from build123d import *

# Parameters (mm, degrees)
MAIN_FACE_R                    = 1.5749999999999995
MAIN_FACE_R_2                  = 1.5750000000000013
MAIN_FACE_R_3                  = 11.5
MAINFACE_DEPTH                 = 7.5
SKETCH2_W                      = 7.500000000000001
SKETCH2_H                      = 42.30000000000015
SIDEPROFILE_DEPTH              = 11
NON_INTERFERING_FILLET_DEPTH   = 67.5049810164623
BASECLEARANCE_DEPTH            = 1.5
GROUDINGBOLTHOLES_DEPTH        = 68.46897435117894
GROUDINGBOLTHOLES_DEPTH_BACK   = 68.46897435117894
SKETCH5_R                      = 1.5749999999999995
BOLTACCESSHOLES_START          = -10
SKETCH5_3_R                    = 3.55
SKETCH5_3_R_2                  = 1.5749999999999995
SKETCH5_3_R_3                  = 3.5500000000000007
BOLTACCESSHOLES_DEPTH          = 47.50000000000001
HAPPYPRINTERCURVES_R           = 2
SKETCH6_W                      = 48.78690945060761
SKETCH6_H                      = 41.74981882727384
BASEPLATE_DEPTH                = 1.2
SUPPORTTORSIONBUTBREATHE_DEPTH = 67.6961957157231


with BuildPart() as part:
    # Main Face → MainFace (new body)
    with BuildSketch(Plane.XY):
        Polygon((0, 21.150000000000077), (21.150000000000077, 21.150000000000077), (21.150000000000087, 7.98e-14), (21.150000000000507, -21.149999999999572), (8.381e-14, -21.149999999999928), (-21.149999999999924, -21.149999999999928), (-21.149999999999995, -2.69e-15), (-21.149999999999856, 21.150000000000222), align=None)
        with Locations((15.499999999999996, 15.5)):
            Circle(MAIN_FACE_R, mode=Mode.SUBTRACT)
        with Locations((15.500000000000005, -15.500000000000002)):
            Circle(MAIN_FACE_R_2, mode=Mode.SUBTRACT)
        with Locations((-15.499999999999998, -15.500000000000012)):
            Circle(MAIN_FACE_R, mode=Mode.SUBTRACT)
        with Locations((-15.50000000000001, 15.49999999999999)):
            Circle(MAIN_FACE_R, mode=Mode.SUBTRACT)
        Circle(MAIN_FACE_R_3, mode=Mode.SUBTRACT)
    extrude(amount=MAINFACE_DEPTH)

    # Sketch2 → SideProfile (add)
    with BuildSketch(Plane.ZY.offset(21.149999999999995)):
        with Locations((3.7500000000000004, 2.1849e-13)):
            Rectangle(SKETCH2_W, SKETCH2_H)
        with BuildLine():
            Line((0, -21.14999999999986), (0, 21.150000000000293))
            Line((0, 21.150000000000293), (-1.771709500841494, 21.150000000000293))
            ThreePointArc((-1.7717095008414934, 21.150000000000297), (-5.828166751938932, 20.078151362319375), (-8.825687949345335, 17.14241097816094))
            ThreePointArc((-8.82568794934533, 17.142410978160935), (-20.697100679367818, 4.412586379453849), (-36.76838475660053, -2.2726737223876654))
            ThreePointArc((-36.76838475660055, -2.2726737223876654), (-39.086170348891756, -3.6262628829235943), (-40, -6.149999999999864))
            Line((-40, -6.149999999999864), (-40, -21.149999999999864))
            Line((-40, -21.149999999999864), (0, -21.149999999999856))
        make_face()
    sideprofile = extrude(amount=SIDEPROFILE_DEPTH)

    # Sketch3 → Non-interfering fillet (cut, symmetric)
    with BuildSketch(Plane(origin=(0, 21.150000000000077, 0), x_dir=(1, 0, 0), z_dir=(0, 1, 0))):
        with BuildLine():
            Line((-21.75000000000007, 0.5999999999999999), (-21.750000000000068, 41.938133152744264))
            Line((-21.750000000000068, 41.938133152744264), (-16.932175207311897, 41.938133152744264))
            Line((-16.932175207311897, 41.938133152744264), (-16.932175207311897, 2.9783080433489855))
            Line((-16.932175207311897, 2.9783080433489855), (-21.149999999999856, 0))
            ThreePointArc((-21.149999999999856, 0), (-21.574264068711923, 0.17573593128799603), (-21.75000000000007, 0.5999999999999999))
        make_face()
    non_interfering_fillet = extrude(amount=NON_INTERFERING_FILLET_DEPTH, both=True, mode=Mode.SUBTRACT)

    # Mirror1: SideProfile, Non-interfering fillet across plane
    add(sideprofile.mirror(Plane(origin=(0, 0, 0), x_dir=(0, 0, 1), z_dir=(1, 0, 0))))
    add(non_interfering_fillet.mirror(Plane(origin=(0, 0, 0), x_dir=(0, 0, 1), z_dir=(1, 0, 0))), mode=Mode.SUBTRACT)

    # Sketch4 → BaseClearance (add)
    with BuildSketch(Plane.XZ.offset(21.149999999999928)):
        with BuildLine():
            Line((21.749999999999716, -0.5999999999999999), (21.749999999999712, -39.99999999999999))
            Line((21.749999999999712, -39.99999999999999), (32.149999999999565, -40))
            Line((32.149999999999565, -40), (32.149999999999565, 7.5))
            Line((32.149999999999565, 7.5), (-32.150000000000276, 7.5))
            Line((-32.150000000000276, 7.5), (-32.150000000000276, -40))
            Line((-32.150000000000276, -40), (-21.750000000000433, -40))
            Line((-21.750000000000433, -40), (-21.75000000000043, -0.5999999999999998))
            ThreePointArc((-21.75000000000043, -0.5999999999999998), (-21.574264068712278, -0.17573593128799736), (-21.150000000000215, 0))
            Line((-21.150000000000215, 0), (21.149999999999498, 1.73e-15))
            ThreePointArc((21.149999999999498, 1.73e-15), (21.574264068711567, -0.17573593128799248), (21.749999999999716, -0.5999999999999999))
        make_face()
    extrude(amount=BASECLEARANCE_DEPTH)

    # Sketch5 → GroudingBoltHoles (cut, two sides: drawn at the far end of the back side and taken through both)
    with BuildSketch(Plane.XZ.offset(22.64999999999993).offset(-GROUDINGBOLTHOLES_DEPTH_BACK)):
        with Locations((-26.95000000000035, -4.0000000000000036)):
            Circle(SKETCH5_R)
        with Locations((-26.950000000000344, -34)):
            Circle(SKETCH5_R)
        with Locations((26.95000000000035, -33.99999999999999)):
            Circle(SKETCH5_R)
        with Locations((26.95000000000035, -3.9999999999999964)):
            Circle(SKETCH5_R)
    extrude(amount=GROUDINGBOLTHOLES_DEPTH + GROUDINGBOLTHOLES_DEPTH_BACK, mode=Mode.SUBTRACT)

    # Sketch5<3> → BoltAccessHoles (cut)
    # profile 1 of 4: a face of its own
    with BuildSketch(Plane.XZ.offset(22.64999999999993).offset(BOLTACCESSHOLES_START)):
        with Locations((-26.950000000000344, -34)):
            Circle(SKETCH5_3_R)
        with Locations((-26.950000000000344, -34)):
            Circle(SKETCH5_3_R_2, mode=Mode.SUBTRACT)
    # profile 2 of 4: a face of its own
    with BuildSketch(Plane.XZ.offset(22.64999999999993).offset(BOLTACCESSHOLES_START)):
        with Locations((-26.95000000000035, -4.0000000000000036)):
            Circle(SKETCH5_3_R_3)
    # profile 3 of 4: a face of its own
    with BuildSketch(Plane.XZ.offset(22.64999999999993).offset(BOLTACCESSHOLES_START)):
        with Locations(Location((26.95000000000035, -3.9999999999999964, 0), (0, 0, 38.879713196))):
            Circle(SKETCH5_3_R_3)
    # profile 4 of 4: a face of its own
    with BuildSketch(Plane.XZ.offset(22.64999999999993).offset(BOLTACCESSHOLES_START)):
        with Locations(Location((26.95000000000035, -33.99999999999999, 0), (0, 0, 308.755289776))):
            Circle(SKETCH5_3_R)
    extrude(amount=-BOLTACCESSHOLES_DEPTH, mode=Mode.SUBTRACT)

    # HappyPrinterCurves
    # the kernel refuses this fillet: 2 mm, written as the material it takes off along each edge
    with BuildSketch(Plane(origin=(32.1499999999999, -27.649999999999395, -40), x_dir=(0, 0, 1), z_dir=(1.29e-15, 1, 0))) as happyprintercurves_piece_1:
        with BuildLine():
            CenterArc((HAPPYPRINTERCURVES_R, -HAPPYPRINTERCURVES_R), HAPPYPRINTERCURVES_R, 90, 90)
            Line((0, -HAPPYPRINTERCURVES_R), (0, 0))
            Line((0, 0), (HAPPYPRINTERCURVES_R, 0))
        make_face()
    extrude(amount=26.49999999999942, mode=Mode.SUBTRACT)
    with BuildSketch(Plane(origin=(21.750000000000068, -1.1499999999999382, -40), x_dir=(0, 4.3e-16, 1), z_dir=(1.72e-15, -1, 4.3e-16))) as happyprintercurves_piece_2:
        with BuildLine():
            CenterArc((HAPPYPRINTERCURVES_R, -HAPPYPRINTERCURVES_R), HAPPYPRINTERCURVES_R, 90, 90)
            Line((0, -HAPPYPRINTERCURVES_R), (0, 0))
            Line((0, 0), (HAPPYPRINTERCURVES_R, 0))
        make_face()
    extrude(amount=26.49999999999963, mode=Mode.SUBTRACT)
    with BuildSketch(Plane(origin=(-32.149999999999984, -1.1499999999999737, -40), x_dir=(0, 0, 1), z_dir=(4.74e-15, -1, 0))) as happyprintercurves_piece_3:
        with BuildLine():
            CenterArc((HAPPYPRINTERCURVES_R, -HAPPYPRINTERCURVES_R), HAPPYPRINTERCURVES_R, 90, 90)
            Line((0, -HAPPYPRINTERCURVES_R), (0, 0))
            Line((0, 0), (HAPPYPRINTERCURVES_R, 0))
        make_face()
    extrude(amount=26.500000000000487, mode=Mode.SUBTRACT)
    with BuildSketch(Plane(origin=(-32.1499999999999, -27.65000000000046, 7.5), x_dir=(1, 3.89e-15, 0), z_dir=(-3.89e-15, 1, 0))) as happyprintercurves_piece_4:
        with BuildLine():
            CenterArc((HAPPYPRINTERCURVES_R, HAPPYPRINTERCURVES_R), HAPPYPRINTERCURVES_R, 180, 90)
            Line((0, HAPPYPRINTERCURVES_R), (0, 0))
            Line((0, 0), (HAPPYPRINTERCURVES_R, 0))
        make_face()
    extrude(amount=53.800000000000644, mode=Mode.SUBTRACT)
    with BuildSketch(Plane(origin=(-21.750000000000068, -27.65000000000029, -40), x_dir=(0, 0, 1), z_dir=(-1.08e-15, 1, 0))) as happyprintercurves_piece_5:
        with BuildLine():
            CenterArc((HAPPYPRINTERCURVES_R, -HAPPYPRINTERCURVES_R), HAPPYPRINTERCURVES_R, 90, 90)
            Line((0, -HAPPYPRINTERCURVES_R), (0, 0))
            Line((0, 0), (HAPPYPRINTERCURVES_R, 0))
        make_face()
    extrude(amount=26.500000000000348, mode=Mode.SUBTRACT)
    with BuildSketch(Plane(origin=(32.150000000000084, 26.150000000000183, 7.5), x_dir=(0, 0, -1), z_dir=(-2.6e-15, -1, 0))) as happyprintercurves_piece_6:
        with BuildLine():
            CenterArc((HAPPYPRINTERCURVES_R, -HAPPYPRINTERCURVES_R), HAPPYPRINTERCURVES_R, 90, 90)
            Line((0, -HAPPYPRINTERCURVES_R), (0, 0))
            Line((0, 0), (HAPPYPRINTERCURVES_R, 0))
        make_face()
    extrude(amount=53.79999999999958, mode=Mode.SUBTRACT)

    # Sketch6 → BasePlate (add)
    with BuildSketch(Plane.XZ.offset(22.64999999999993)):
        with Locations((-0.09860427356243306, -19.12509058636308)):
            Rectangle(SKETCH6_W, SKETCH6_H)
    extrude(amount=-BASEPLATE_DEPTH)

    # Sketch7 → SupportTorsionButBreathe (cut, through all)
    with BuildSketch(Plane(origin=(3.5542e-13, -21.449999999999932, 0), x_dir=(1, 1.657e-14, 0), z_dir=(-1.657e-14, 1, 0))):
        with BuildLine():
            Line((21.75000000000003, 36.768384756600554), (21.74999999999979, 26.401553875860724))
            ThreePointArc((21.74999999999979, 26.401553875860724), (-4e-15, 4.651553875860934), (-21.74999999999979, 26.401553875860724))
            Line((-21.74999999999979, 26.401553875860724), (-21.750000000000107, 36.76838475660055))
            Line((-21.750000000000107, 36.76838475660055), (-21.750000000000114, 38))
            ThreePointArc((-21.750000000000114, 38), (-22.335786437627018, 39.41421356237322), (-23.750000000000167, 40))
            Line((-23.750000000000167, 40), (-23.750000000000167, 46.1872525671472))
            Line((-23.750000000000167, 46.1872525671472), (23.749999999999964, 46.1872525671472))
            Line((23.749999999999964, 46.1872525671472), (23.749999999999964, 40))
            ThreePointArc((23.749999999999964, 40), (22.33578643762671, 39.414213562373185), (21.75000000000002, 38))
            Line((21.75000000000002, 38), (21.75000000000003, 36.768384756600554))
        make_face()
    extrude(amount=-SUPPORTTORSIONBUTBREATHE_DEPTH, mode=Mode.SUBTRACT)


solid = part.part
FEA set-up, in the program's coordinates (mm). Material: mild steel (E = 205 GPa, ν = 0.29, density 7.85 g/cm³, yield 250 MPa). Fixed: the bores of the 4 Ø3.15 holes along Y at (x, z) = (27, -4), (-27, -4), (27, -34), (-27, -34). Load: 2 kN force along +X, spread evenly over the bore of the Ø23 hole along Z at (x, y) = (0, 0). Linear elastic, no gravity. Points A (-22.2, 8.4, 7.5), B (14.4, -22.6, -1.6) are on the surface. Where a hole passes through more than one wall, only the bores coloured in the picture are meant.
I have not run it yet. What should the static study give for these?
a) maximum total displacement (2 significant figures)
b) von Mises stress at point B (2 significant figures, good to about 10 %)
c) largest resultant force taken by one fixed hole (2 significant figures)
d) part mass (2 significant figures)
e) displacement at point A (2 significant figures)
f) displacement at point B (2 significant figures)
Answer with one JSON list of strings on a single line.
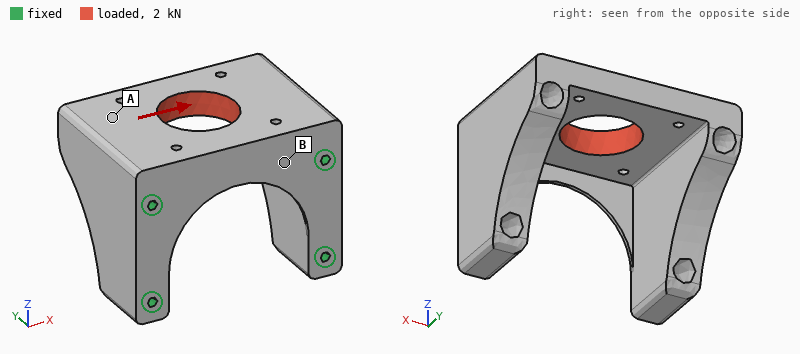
["4.4 µm", "14 MPa", "1.2 kN", "310 g", "3.5 µm", "0.92 µm"]
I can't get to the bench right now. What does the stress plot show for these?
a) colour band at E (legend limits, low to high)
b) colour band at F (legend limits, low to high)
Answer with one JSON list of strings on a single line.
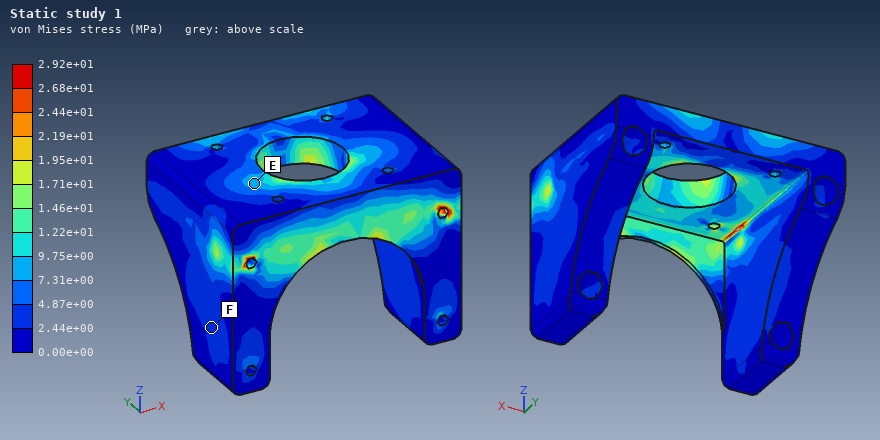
["7.31e+00 to 9.75e+00 MPa", "2.44e+00 to 4.87e+00 MPa"]
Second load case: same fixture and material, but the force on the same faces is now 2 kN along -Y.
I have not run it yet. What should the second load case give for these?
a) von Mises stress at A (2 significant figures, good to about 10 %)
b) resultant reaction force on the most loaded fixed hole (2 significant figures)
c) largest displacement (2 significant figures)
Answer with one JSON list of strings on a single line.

["4.4 MPa", "1.2 kN", "3.3 µm"]
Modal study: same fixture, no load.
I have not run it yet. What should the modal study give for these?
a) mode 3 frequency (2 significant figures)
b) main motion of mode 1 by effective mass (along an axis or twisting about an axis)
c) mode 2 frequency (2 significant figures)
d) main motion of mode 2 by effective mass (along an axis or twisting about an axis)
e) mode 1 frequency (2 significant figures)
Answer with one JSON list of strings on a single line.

["14 kHz", "along Z", "9100 Hz", "along X", "8700 Hz"]
